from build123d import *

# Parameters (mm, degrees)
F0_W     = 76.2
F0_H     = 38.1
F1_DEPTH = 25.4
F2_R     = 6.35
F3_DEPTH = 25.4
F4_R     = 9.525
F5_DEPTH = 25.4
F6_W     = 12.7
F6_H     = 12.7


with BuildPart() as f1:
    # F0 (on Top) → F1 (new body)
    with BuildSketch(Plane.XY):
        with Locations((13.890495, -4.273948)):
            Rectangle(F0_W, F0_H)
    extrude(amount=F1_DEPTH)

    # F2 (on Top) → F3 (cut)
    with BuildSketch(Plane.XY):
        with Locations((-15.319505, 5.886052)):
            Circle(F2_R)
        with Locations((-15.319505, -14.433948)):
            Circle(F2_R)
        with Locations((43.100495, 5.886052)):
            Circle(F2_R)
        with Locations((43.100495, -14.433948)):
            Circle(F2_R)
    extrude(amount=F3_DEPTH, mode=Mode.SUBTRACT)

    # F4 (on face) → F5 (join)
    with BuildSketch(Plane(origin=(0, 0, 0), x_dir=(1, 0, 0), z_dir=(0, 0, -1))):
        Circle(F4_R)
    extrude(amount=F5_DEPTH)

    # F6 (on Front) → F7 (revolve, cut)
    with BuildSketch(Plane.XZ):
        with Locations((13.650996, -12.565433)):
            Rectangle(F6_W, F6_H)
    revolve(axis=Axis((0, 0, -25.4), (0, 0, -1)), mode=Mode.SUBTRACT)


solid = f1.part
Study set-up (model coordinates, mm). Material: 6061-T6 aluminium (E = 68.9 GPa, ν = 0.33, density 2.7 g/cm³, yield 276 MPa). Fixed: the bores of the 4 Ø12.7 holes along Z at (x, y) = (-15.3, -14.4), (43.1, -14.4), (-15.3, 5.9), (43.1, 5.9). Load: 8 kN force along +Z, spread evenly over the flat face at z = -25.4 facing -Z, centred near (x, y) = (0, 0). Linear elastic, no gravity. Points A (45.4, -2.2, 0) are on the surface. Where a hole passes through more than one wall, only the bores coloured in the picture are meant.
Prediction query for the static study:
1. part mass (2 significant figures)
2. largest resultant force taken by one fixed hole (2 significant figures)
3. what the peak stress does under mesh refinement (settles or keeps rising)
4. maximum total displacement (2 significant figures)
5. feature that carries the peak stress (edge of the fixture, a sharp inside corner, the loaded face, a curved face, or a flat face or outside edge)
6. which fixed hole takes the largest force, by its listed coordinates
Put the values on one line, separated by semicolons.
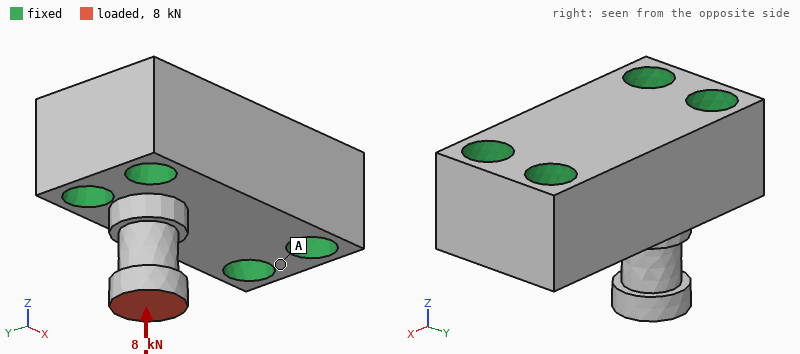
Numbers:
180 g; 4.3 kN; keeps rising; 23 µm; edge of the fixture; (-15.3, 5.9)
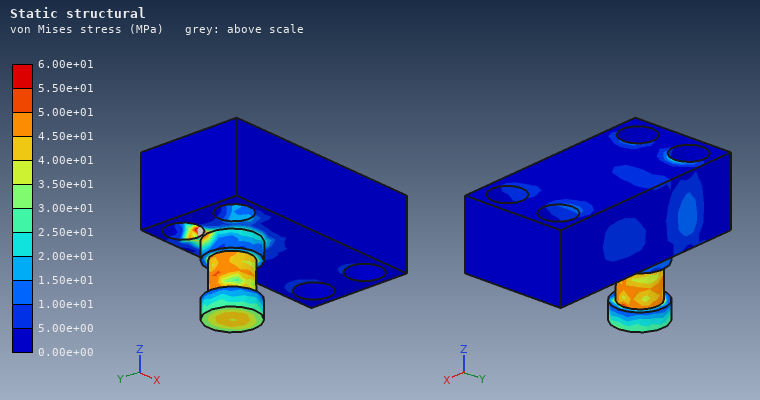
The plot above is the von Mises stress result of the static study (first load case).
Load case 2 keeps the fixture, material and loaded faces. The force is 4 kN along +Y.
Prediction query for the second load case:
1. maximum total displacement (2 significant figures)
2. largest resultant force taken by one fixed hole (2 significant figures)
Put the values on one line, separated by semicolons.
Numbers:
0.17 mm; 4.6 kN
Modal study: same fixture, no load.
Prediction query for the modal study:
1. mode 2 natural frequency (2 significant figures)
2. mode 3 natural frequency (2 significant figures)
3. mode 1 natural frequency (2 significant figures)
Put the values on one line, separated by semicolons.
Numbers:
12 kHz; 24 kHz; 12 kHz
